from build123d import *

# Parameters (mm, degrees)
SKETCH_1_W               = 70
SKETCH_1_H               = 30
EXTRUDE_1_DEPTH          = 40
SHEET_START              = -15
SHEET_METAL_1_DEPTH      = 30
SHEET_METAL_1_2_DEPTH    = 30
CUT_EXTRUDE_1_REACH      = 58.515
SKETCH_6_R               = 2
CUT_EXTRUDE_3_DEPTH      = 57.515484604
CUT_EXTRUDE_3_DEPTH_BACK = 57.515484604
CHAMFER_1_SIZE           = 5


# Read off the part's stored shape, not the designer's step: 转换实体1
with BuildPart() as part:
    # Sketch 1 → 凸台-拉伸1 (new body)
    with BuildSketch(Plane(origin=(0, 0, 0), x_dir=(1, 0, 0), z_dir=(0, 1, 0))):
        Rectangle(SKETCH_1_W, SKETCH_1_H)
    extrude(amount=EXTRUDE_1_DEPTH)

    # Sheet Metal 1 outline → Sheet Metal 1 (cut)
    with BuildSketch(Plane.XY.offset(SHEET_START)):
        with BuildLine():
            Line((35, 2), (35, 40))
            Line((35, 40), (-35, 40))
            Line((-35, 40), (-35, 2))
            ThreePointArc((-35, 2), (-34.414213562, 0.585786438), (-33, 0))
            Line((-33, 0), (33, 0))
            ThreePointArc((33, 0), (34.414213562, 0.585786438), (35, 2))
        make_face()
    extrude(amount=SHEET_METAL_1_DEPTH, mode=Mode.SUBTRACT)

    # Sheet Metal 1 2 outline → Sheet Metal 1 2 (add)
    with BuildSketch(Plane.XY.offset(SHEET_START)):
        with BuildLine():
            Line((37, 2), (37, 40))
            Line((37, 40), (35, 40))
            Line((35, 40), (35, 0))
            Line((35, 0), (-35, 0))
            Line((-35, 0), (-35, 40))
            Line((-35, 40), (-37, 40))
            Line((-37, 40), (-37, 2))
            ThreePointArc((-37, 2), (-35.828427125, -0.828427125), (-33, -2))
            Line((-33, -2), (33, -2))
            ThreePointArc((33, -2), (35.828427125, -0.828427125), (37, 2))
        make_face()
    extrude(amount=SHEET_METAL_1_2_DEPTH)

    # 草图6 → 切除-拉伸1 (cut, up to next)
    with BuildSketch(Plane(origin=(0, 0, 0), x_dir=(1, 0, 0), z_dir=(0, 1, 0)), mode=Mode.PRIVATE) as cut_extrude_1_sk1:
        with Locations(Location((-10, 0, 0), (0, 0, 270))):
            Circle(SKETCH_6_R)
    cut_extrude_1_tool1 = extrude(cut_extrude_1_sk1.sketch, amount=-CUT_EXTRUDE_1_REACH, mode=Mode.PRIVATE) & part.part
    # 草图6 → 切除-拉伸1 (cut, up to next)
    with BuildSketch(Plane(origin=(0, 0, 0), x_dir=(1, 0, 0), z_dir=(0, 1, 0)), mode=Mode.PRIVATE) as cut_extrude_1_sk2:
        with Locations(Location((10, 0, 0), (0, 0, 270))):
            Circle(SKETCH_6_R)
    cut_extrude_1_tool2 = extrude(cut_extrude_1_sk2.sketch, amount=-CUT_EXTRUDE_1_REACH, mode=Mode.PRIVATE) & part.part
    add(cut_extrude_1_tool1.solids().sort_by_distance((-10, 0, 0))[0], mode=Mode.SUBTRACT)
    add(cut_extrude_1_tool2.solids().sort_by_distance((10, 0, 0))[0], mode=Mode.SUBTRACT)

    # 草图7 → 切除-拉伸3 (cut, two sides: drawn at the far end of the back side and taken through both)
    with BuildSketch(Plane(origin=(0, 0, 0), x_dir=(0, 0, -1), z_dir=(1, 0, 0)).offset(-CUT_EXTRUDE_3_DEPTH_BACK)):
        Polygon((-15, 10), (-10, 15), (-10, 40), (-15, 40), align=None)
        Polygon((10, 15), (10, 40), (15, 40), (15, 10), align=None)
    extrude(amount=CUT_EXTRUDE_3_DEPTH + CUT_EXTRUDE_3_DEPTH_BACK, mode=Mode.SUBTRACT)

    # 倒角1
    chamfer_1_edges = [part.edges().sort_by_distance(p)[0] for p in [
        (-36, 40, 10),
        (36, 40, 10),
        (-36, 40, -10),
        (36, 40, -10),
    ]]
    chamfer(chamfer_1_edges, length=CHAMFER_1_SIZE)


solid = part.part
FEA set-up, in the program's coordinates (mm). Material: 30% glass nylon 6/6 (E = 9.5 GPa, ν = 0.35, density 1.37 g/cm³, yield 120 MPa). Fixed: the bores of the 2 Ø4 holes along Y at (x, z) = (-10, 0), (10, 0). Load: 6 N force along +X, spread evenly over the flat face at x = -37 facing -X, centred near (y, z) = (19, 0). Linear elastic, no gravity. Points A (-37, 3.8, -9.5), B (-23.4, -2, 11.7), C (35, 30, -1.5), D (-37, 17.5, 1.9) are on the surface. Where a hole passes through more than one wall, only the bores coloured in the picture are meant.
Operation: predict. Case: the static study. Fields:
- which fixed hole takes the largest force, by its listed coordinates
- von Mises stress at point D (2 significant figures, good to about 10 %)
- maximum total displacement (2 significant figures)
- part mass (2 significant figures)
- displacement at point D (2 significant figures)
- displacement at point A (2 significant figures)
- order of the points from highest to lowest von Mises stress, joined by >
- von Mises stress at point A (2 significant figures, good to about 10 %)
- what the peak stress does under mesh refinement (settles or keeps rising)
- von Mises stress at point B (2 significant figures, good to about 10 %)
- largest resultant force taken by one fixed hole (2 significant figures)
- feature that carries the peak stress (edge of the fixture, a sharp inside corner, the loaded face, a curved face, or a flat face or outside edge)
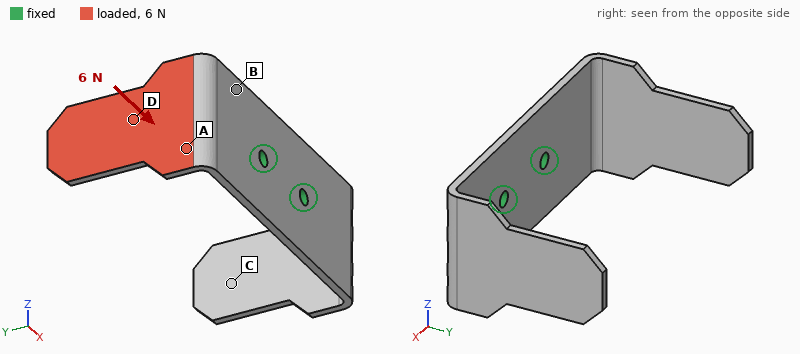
(-10, 0)
2.2 MPa
0.90 mm
11 g
0.41 mm
0.23 mm
B > A > D > C
3.9 MPa
keeps rising
5.7 MPa
4.9 N
edge of the fixture
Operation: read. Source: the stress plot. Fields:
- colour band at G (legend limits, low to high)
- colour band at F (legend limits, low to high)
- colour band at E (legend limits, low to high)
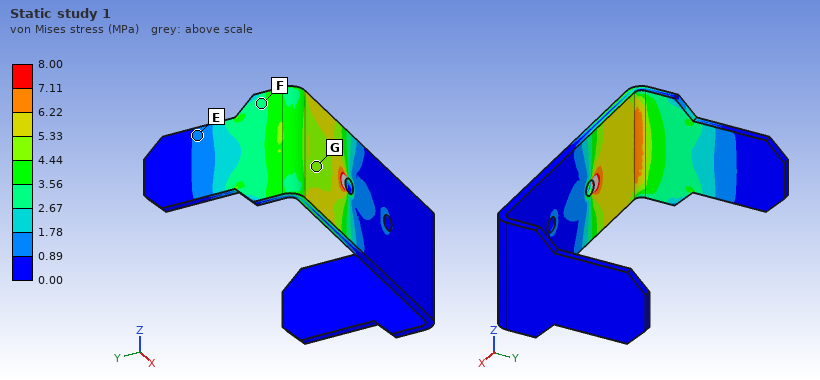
4.44 to 5.33 MPa
2.67 to 3.56 MPa
0.89 to 1.78 MPa
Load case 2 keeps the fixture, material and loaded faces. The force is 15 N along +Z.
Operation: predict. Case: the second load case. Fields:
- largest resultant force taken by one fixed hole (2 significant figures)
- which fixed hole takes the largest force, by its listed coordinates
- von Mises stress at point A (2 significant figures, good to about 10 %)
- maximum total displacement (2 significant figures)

31 N
(-10, 0)
4.6 MPa
0.99 mm
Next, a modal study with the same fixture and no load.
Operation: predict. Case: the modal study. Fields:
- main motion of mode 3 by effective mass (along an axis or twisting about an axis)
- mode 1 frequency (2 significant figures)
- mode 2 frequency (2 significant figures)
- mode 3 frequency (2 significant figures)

twisting about Y
310 Hz
310 Hz
480 Hz
